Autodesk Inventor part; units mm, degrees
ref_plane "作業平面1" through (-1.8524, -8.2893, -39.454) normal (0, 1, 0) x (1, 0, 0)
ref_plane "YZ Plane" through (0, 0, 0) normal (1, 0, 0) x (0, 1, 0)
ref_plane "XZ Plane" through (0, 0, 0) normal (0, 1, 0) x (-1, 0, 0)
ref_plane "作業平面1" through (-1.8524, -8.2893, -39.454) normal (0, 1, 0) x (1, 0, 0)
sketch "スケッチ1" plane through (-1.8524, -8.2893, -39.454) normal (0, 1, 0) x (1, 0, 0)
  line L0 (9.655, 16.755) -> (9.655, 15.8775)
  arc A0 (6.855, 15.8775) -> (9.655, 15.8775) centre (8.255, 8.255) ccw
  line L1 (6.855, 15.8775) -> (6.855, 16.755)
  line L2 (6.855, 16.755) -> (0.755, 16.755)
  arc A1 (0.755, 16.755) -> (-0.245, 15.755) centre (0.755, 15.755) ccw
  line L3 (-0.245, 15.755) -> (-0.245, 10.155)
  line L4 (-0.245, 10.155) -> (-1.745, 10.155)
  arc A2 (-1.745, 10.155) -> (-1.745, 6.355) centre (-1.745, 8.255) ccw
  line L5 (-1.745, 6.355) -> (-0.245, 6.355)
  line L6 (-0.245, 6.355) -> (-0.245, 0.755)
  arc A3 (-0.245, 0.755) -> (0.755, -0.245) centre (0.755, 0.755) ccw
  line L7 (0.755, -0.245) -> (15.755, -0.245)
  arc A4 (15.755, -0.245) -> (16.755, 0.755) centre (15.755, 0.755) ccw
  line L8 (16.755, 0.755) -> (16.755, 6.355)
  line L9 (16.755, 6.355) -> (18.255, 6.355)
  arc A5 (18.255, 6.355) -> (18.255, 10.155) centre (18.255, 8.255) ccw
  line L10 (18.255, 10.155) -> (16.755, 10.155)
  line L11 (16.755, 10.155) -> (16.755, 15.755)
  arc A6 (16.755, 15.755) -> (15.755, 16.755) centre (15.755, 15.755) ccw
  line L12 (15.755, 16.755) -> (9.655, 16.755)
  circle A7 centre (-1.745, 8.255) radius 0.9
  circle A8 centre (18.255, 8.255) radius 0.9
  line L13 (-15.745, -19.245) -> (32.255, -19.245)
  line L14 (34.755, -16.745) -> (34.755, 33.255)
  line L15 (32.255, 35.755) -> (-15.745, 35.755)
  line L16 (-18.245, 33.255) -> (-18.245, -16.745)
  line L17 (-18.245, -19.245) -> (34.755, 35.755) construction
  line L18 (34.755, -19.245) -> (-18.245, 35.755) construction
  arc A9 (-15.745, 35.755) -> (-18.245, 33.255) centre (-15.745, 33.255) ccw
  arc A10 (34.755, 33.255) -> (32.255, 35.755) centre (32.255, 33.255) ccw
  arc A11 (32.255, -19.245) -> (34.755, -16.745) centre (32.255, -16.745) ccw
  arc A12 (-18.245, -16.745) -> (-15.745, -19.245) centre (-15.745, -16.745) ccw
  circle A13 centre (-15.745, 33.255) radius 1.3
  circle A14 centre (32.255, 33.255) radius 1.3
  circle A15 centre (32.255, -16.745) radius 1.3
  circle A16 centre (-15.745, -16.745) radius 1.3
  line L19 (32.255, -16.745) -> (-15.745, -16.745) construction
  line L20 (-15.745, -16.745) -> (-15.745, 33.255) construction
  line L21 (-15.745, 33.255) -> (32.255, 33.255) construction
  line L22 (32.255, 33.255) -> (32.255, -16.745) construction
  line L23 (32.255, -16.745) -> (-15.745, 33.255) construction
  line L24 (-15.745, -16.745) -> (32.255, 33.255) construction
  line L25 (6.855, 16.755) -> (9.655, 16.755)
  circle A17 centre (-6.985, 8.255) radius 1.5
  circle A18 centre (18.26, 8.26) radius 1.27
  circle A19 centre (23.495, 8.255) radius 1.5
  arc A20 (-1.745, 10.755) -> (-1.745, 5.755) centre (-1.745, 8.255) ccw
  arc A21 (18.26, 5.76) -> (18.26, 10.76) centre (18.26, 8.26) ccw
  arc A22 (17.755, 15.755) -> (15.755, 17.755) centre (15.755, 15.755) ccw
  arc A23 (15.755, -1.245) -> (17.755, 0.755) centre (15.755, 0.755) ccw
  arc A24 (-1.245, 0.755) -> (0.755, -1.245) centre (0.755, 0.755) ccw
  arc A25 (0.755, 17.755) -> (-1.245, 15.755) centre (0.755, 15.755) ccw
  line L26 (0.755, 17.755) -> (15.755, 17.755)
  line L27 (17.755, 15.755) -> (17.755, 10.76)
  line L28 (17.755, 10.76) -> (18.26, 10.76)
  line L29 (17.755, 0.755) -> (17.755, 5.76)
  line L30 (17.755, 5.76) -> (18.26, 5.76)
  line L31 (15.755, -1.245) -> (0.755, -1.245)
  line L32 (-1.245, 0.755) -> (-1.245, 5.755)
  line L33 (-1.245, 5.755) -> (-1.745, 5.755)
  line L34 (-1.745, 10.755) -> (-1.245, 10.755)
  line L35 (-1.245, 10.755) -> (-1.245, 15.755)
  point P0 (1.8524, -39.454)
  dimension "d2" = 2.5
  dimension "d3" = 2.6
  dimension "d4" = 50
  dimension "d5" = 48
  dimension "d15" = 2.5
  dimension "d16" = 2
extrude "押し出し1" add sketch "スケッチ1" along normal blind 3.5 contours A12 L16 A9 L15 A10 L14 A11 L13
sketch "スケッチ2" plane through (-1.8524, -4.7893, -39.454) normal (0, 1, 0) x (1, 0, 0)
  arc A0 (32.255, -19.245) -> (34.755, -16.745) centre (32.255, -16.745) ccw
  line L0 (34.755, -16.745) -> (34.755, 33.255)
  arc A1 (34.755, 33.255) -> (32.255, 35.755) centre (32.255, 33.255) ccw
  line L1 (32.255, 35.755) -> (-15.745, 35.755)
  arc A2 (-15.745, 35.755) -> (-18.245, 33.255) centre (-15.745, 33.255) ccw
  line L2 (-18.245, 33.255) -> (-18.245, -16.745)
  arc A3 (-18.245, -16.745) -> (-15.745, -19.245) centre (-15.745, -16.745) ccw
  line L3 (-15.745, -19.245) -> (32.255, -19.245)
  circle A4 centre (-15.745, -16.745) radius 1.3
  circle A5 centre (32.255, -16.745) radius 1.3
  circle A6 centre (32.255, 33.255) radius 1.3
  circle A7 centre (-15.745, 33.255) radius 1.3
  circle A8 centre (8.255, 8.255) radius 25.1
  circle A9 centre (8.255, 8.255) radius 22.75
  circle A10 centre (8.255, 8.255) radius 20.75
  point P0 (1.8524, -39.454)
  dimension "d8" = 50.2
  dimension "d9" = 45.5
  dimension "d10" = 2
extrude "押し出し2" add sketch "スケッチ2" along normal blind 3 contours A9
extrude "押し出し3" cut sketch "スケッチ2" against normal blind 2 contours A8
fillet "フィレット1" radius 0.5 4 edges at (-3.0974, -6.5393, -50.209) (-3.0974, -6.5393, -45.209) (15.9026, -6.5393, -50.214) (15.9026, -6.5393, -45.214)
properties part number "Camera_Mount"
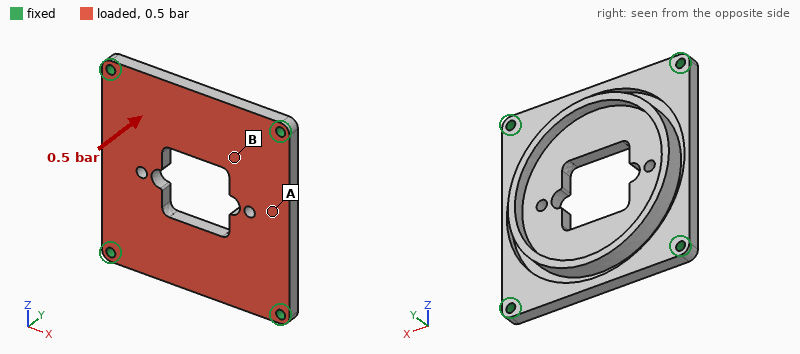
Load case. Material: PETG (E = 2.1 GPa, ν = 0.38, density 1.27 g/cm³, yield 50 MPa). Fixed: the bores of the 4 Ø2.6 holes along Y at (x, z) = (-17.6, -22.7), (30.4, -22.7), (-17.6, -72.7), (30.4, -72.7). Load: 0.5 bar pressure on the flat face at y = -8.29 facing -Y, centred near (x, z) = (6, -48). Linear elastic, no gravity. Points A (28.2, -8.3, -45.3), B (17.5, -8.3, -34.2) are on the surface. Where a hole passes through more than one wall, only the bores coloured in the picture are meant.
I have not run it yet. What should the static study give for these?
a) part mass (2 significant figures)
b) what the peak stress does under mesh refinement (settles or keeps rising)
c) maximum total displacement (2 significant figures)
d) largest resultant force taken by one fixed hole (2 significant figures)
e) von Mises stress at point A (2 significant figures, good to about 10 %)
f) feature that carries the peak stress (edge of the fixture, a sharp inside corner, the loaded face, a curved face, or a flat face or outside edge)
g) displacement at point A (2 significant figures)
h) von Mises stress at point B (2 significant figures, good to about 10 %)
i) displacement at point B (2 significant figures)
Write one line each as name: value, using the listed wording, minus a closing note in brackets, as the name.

part mass: 11 g
what the peak stress does under mesh refinement: keeps rising
maximum total displacement: 0.26 mm
largest resultant force taken by one fixed hole: 33 N
von Mises stress at point A: 3.0 MPa
feature that carries the peak stress: edge of the fixture
displacement at point A: 0.18 mm
von Mises stress at point B: 1.4 MPa
displacement at point B: 0.19 mm
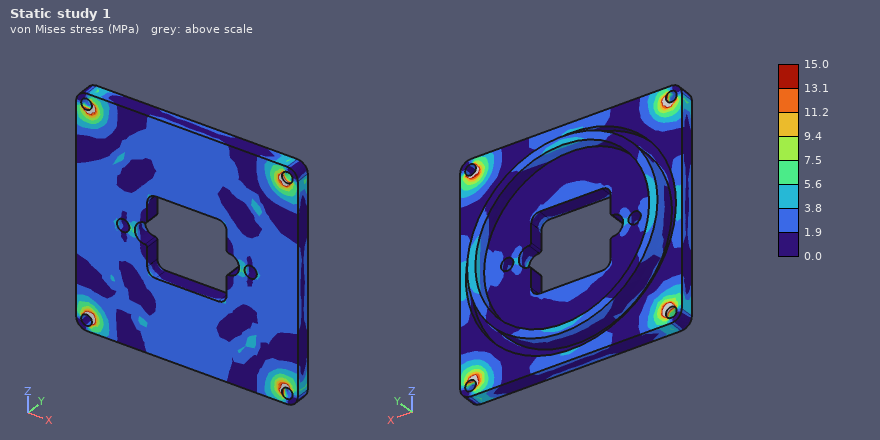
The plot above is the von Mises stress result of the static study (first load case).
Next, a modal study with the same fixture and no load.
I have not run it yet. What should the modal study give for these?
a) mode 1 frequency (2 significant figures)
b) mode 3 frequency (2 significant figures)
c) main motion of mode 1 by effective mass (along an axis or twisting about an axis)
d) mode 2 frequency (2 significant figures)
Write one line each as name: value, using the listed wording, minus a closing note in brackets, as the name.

mode 1 frequency: 1300 Hz
mode 3 frequency: 1800 Hz
main motion of mode 1 by effective mass: along Y
mode 2 frequency: 1800 Hz
